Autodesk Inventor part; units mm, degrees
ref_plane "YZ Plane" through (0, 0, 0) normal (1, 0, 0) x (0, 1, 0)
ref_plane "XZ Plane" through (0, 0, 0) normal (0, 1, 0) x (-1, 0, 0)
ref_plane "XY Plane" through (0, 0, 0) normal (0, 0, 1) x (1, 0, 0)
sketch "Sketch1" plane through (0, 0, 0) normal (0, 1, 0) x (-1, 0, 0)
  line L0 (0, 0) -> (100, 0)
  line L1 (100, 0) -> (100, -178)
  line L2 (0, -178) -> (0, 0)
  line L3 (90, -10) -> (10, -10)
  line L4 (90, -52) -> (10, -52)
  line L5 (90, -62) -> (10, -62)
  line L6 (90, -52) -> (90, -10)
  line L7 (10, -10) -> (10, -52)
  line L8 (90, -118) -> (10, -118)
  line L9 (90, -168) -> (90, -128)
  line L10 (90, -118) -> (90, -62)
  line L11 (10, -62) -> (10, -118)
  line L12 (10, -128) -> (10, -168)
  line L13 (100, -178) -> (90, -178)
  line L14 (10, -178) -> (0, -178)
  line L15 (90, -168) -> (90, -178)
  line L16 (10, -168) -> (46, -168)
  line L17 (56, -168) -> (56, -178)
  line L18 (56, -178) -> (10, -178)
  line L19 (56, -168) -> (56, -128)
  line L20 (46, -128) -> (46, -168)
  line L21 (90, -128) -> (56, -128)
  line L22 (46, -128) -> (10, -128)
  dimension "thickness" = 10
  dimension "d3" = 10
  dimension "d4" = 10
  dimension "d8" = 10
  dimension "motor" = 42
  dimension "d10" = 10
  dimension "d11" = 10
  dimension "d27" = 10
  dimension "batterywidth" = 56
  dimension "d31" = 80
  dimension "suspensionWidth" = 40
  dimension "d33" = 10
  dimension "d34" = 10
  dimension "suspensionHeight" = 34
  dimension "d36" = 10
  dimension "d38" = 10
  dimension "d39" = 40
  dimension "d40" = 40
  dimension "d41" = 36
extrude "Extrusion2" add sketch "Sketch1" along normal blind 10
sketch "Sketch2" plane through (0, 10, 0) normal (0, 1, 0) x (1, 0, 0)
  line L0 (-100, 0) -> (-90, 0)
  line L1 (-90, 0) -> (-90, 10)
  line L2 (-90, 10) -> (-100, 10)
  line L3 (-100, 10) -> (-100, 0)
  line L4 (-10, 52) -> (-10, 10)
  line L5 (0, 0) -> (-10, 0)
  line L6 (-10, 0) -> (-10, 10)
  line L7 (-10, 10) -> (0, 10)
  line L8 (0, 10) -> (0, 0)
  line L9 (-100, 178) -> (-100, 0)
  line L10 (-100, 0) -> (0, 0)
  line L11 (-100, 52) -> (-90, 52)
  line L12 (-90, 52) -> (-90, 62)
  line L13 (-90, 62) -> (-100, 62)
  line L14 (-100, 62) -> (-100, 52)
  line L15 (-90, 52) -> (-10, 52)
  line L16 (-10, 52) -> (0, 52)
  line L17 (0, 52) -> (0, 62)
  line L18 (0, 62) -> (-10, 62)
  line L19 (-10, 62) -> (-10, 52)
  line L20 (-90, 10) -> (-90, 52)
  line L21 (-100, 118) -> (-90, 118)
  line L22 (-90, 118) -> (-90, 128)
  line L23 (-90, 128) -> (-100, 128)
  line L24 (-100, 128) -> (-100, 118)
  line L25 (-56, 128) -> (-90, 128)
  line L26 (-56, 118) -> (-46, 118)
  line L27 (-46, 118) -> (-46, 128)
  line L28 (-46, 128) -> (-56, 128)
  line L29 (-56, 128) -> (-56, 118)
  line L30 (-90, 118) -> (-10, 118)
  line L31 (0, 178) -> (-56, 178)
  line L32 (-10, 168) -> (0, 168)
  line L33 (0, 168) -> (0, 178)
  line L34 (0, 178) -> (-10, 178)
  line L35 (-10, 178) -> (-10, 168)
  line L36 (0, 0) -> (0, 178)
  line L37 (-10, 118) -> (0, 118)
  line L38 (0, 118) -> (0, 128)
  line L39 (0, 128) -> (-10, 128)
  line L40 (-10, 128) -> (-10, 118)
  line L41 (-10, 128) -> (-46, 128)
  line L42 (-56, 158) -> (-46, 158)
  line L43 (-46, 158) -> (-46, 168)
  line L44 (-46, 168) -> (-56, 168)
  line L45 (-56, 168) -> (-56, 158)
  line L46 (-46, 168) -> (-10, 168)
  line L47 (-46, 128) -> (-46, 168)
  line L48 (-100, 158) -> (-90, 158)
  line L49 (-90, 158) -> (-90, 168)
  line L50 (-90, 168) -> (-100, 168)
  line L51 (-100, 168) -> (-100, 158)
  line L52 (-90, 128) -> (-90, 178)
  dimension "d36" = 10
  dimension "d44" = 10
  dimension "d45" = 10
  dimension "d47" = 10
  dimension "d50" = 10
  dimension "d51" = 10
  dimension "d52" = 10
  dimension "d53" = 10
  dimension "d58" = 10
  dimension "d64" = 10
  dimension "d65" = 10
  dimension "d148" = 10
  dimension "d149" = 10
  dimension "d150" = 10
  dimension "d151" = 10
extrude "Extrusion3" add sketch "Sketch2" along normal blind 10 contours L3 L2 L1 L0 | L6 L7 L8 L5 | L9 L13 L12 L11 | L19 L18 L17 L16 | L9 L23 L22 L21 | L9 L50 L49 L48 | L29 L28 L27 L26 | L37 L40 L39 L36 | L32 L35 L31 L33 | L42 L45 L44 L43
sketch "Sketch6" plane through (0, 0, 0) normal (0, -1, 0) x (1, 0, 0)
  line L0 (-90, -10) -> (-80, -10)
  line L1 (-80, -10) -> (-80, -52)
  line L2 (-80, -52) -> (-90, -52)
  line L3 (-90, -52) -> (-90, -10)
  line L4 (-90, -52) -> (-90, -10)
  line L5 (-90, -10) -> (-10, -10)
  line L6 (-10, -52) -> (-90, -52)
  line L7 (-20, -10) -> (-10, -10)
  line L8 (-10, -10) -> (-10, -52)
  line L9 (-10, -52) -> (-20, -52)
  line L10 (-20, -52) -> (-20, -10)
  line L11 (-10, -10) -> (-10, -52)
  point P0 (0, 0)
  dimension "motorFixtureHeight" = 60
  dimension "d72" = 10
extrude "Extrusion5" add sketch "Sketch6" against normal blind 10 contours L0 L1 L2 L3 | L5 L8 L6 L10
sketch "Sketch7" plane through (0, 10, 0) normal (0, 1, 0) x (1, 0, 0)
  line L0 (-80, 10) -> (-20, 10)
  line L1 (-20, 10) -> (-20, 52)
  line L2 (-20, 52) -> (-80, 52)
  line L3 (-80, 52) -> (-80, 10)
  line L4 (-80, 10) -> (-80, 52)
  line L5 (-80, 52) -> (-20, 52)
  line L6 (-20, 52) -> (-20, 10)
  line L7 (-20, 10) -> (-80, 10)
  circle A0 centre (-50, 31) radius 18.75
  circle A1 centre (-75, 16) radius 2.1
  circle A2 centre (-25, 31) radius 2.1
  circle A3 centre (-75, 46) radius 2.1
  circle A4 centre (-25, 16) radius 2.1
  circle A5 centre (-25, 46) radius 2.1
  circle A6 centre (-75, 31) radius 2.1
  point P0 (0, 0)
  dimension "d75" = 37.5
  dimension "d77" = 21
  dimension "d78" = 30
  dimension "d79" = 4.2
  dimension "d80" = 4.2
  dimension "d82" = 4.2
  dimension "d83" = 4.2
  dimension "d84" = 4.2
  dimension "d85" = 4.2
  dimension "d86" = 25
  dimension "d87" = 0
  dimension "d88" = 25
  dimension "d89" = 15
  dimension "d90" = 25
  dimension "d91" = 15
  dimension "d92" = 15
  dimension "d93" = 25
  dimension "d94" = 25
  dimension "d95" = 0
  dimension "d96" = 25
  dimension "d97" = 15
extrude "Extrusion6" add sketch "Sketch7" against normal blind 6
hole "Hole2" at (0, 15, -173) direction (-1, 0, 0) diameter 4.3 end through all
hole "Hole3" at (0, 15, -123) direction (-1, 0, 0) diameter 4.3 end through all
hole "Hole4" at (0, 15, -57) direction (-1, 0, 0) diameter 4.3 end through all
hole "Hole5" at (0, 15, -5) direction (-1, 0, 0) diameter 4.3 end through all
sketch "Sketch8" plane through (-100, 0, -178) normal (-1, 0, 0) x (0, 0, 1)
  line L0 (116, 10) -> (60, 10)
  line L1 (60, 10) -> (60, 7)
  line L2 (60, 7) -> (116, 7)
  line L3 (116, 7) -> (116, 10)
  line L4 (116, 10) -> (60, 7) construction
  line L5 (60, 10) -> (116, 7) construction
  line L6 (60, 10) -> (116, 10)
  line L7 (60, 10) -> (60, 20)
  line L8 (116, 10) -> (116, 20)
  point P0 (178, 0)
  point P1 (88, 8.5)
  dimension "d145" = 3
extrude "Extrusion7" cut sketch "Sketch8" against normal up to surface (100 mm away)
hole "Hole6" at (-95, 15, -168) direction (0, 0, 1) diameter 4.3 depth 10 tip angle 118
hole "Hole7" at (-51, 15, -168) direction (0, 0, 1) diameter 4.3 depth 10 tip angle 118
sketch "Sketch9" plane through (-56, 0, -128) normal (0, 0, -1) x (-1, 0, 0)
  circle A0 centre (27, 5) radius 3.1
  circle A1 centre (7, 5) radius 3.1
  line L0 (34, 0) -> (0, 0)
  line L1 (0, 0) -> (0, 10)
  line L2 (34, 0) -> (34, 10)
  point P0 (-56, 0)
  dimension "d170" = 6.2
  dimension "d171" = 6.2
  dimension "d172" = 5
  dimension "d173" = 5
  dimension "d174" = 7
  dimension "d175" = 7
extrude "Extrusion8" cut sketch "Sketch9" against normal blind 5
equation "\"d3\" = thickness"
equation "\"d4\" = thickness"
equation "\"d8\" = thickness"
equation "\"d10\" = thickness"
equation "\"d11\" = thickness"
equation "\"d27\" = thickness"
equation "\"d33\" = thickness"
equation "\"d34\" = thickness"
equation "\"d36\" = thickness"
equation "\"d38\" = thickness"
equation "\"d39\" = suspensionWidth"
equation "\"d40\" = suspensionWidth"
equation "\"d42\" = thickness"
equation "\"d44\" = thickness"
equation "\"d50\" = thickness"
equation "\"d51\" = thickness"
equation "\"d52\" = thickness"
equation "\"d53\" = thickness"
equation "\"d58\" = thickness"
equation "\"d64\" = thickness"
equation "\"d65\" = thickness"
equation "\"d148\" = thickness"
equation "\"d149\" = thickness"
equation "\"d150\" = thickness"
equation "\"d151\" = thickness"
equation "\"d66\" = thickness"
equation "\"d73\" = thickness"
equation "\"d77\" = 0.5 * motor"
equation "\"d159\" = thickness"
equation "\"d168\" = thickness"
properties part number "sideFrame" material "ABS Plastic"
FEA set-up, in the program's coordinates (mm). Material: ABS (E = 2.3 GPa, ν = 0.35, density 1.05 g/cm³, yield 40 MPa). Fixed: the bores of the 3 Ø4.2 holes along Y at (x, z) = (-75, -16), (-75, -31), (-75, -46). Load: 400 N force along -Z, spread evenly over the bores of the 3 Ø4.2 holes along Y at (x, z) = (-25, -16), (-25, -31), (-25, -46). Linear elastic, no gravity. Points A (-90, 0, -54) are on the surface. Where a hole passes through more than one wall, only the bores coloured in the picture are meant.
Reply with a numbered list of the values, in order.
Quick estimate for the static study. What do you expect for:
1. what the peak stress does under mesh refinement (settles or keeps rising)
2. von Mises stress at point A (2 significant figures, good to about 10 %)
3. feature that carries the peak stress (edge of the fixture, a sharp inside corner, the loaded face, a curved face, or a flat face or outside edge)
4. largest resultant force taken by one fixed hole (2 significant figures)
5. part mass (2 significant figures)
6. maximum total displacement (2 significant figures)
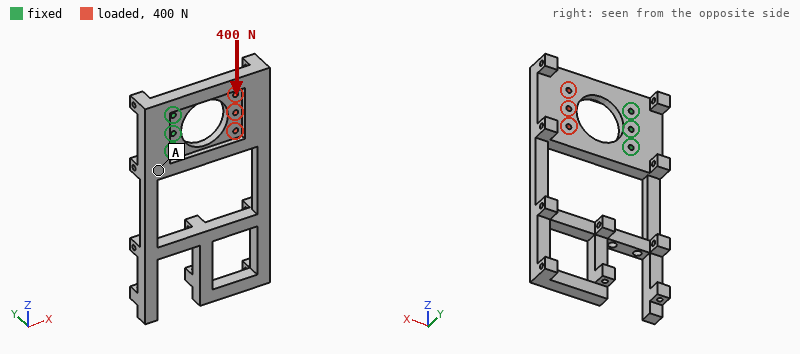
1. keeps rising
2. 2.0 MPa
3. edge of the fixture
4. 590 N
5. 94 g
6. 1.2 mm
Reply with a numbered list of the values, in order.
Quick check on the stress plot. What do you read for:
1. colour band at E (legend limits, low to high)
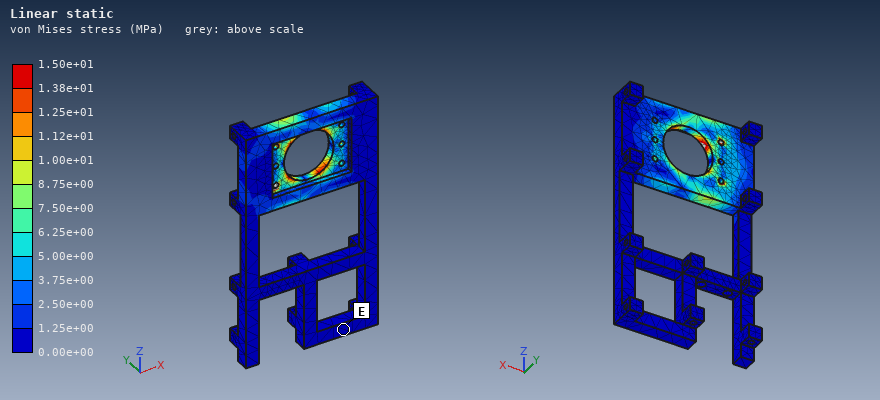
1. 0.00e+00 to 1.25e+00 MPa
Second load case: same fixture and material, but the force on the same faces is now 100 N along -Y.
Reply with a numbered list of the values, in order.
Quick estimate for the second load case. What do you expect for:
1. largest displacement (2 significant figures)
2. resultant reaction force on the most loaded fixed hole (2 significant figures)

1. 2.2 mm
2. 80 N
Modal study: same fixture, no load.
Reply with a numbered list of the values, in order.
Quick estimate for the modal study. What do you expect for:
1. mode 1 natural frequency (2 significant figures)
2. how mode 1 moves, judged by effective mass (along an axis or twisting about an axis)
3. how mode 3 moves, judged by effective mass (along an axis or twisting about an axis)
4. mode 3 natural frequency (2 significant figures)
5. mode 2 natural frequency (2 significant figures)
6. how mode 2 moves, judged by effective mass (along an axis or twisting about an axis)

1. 54 Hz
2. along Y
3. along X
4. 200 Hz
5. 140 Hz
6. twisting about Z
